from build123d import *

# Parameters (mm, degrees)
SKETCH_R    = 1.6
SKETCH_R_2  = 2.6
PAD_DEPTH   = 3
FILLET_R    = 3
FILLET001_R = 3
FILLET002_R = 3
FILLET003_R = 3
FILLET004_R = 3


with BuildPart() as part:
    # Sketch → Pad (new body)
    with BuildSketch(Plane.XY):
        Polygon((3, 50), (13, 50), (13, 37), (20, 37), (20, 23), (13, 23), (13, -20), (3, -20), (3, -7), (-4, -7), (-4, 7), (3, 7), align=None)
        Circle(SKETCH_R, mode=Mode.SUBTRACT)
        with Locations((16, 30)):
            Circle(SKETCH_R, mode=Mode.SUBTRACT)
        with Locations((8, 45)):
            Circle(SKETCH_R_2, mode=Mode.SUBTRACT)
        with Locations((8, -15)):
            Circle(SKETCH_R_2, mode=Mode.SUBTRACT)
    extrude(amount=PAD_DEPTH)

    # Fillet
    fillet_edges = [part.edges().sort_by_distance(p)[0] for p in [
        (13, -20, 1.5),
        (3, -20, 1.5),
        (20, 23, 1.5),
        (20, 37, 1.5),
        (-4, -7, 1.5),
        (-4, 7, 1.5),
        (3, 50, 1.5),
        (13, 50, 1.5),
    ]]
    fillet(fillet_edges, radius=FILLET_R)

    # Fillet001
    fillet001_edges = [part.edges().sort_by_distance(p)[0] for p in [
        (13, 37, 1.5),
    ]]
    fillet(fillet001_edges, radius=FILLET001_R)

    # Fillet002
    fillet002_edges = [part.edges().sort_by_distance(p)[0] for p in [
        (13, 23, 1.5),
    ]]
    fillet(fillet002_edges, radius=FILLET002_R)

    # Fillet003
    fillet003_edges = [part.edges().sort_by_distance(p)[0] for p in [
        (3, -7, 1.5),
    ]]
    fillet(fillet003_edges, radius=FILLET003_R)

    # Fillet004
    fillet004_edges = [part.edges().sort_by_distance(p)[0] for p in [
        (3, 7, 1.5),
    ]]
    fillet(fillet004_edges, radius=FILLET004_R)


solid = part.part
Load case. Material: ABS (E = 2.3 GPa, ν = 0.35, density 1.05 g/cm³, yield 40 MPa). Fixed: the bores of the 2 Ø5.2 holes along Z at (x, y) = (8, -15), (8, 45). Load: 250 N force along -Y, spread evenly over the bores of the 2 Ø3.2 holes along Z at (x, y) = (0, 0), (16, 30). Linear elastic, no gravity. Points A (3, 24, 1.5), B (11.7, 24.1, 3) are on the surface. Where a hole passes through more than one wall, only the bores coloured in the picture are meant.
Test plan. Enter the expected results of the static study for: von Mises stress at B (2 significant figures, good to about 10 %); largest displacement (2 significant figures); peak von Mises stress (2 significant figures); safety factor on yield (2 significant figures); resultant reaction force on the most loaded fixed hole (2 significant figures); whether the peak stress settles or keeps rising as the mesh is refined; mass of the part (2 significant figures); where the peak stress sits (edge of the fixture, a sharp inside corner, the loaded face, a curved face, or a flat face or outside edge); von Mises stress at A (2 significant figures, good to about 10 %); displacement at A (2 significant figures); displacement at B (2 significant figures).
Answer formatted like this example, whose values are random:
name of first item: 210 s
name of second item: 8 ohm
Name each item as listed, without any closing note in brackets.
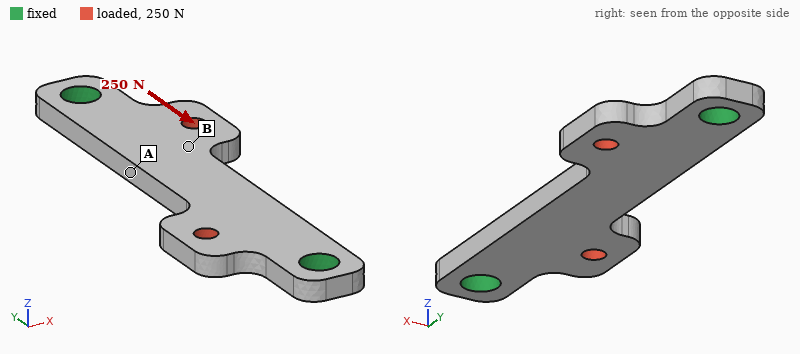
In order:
von Mises stress at B: 3.2 MPa
largest displacement: 0.20 mm
peak von Mises stress: 20 MPa
safety factor on yield: 2.0
resultant reaction force on the most loaded fixed hole: 130 N
whether the peak stress settles or keeps rising as the mesh is refined: settles
mass of the part: 2.6 g
where the peak stress sits: a curved face
von Mises stress at A: 7.1 MPa
displacement at A: 0.15 mm
displacement at B: 0.16 mm
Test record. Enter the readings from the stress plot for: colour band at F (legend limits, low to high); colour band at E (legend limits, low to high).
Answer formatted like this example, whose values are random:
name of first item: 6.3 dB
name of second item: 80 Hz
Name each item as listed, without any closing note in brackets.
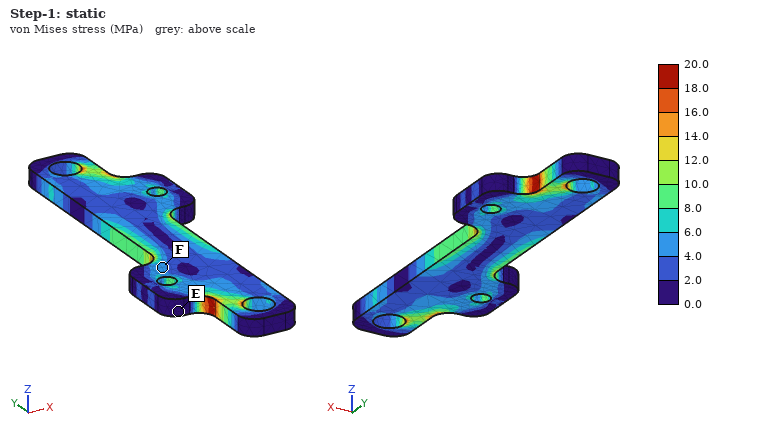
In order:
colour band at F: 4.0 to 6.0 MPa
colour band at E: 0.0 to 2.0 MPa
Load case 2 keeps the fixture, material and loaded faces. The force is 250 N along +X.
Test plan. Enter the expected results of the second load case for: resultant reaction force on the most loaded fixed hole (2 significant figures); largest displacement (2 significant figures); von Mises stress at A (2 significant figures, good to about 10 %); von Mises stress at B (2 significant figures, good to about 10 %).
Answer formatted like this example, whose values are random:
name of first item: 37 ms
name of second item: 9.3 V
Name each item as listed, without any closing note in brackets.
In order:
resultant reaction force on the most loaded fixed hole: 130 N
largest displacement: 0.32 mm
von Mises stress at A: 10 MPa
von Mises stress at B: 4.7 MPa
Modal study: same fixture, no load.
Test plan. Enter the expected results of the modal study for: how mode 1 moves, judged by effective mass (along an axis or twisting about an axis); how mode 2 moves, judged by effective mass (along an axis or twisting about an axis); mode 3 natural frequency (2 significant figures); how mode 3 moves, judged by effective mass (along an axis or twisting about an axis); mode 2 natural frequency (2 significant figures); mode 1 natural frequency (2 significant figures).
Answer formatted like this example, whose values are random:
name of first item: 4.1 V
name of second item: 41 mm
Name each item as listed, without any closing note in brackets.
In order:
how mode 1 moves, judged by effective mass: along Z
how mode 2 moves, judged by effective mass: twisting about Y
mode 3 natural frequency: 3200 Hz
how mode 3 moves, judged by effective mass: along X
mode 2 natural frequency: 2300 Hz
mode 1 natural frequency: 1300 Hz
